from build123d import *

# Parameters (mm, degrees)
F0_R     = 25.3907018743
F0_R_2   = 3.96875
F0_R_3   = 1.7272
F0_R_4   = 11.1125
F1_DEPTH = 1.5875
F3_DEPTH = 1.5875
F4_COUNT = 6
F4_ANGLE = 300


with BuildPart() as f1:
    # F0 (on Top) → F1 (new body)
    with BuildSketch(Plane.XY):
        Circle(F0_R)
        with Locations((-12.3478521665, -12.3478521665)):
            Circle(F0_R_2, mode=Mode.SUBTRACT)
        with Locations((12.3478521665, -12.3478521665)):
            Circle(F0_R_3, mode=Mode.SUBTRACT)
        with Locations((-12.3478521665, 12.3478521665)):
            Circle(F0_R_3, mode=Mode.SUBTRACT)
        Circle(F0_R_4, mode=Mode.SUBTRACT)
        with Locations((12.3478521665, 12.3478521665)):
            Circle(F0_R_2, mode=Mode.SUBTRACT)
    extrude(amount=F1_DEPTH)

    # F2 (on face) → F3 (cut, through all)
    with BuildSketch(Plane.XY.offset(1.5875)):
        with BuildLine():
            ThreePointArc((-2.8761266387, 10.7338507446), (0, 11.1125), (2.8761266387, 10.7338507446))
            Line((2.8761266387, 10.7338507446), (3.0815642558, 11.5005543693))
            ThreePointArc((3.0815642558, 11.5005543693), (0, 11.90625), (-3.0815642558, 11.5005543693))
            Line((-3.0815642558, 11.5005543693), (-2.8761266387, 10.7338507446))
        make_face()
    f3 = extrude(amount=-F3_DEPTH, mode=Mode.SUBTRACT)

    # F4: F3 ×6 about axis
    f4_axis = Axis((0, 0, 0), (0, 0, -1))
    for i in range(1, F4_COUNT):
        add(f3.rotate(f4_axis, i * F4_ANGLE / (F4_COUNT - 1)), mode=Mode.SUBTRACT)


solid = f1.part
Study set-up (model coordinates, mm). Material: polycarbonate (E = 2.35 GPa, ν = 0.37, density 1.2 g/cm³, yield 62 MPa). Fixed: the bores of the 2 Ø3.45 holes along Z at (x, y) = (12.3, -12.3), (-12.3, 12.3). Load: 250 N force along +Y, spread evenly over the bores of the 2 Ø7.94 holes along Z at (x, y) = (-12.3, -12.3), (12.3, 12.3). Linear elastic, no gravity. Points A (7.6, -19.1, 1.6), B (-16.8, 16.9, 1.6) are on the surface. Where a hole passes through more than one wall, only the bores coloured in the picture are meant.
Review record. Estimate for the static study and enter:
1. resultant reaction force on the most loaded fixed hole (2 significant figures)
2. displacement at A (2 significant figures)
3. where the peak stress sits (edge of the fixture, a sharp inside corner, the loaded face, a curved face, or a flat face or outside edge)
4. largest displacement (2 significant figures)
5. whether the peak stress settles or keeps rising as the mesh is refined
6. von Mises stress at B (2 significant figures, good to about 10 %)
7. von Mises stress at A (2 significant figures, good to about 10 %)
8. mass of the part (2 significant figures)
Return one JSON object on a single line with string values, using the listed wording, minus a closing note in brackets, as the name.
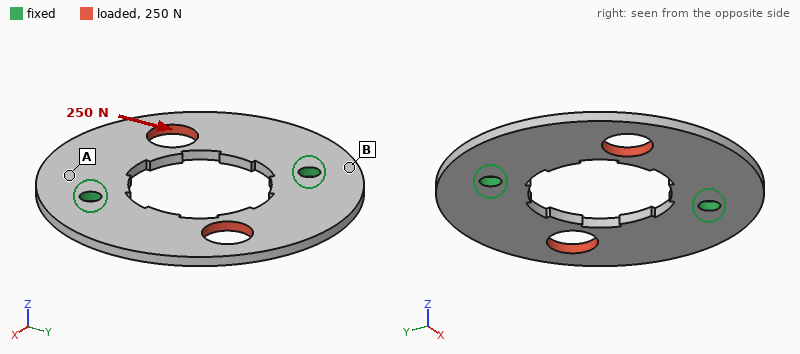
{"resultant reaction force on the most loaded fixed hole": "130 N", "displacement at A": "0.025 mm", "where the peak stress sits": "a sharp inside corner", "largest displacement": "0.12 mm", "whether the peak stress settles or keeps rising as the mesh is refined": "keeps rising", "von Mises stress at B": "5.8 MPa", "von Mises stress at A": "2.8 MPa", "mass of the part": "2.8 g"}
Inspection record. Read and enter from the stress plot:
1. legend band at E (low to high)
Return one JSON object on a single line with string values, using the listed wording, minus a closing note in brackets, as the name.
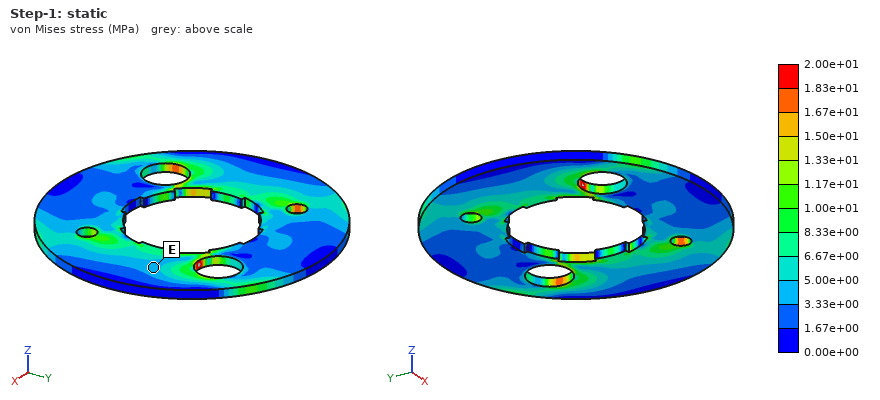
{"legend band at E": "3.33e+00 to 5.00e+00 MPa"}
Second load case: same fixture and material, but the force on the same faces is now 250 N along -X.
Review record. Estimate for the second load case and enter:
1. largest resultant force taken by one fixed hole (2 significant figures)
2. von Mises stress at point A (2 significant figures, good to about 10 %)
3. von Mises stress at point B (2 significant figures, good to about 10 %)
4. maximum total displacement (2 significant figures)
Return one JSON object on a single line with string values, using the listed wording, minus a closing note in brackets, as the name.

{"largest resultant force taken by one fixed hole": "130 N", "von Mises stress at point A": "4.5 MPa", "von Mises stress at point B": "5.9 MPa", "maximum total displacement": "0.12 mm"}
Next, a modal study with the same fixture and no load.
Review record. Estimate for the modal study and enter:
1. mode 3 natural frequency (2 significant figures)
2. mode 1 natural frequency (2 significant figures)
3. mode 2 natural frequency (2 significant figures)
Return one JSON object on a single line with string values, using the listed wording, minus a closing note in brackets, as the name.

{"mode 3 natural frequency": "1400 Hz", "mode 1 natural frequency": "590 Hz", "mode 2 natural frequency": "590 Hz"}
